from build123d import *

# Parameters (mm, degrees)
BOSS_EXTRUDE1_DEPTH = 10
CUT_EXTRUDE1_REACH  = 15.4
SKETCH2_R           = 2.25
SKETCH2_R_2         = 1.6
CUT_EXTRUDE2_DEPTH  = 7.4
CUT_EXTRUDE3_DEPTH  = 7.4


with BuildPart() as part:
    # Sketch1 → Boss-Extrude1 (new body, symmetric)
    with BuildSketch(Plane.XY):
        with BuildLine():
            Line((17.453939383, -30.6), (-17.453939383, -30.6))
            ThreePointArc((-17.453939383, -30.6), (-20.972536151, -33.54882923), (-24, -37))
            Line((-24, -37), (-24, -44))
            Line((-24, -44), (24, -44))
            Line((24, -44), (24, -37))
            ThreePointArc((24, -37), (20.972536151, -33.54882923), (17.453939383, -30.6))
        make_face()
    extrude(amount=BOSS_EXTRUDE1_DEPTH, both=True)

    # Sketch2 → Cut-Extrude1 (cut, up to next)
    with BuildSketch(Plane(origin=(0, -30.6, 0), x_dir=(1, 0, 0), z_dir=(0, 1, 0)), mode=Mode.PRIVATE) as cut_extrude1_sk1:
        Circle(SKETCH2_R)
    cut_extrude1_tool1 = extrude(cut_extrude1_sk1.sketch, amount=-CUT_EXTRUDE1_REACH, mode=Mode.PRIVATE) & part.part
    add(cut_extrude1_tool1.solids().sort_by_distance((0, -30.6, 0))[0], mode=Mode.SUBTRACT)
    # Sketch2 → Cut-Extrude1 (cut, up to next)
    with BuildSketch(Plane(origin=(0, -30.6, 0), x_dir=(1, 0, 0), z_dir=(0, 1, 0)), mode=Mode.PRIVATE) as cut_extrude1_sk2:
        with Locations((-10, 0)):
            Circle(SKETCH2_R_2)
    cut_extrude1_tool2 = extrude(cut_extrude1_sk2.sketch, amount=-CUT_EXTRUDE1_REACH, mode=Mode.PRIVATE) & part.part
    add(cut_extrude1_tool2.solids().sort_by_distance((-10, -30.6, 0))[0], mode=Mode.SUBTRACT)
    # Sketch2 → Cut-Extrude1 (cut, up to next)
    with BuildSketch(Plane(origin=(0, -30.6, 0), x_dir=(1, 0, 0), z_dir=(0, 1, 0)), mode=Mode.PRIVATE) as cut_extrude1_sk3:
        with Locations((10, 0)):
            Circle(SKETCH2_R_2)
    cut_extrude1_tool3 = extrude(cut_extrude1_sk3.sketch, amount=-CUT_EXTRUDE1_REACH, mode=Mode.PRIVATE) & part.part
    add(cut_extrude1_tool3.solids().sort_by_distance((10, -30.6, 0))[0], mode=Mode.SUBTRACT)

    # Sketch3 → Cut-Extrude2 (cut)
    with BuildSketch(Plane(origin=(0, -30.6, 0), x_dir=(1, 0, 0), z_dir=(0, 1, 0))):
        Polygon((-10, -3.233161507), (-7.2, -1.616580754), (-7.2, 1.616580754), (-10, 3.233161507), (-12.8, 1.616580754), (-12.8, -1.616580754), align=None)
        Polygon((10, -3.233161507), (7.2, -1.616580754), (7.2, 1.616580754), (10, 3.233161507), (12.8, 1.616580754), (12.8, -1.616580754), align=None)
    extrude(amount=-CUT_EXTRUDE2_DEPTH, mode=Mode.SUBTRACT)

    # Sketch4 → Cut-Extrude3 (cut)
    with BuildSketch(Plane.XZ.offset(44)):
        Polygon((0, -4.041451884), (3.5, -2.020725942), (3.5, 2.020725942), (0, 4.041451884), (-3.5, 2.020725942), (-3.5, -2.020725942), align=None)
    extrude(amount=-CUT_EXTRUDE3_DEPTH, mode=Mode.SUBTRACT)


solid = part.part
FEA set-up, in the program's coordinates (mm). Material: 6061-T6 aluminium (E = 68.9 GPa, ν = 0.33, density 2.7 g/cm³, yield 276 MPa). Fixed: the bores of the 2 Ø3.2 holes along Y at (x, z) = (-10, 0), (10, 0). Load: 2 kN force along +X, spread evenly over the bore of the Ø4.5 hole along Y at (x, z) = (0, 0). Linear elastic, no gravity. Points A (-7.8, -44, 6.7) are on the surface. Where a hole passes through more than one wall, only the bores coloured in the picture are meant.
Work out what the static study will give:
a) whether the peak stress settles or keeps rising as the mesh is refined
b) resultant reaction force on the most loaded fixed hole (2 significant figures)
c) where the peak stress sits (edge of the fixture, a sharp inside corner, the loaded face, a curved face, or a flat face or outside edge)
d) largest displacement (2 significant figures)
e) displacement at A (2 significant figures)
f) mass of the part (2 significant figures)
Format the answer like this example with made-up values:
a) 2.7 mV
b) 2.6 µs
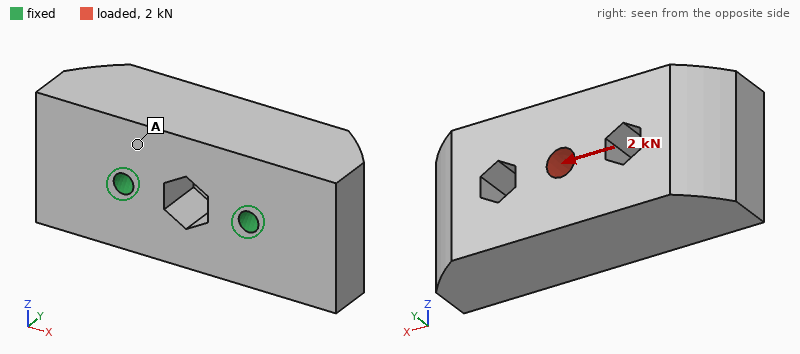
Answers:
a) keeps rising
b) 1.2 kN
c) edge of the fixture
d) 5.2 µm
e) 0.95 µm
f) 30 g
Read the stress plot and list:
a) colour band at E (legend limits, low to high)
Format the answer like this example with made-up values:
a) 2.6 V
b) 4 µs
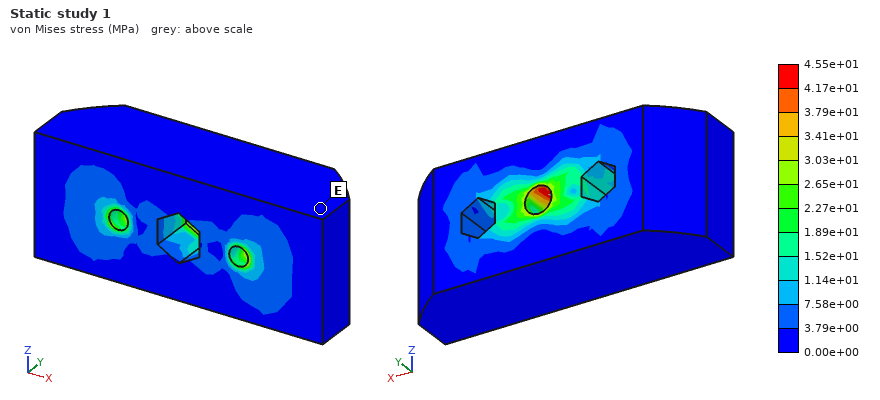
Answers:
a) 0.00e+00 to 3.79e+00 MPa
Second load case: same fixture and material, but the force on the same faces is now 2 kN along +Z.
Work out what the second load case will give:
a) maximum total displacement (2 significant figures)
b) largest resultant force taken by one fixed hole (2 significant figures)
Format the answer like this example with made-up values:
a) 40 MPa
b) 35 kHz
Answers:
a) 18 µm
b) 1.0 kN
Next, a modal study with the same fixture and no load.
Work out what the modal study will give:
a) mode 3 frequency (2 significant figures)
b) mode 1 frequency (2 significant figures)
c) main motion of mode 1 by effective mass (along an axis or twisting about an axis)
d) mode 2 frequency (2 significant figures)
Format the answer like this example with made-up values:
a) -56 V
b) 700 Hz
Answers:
a) 20 kHz
b) 14 kHz
c) along Z
d) 20 kHz
